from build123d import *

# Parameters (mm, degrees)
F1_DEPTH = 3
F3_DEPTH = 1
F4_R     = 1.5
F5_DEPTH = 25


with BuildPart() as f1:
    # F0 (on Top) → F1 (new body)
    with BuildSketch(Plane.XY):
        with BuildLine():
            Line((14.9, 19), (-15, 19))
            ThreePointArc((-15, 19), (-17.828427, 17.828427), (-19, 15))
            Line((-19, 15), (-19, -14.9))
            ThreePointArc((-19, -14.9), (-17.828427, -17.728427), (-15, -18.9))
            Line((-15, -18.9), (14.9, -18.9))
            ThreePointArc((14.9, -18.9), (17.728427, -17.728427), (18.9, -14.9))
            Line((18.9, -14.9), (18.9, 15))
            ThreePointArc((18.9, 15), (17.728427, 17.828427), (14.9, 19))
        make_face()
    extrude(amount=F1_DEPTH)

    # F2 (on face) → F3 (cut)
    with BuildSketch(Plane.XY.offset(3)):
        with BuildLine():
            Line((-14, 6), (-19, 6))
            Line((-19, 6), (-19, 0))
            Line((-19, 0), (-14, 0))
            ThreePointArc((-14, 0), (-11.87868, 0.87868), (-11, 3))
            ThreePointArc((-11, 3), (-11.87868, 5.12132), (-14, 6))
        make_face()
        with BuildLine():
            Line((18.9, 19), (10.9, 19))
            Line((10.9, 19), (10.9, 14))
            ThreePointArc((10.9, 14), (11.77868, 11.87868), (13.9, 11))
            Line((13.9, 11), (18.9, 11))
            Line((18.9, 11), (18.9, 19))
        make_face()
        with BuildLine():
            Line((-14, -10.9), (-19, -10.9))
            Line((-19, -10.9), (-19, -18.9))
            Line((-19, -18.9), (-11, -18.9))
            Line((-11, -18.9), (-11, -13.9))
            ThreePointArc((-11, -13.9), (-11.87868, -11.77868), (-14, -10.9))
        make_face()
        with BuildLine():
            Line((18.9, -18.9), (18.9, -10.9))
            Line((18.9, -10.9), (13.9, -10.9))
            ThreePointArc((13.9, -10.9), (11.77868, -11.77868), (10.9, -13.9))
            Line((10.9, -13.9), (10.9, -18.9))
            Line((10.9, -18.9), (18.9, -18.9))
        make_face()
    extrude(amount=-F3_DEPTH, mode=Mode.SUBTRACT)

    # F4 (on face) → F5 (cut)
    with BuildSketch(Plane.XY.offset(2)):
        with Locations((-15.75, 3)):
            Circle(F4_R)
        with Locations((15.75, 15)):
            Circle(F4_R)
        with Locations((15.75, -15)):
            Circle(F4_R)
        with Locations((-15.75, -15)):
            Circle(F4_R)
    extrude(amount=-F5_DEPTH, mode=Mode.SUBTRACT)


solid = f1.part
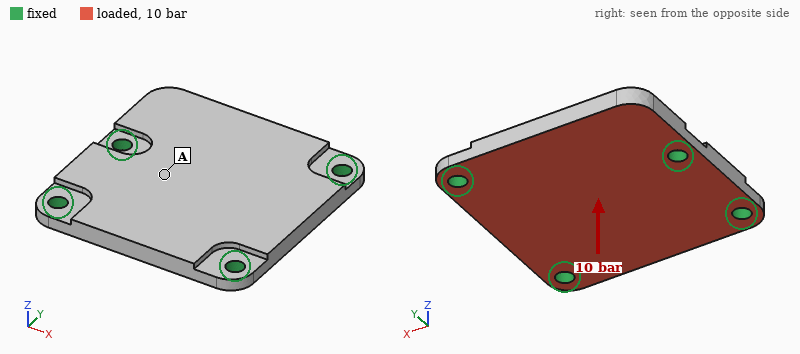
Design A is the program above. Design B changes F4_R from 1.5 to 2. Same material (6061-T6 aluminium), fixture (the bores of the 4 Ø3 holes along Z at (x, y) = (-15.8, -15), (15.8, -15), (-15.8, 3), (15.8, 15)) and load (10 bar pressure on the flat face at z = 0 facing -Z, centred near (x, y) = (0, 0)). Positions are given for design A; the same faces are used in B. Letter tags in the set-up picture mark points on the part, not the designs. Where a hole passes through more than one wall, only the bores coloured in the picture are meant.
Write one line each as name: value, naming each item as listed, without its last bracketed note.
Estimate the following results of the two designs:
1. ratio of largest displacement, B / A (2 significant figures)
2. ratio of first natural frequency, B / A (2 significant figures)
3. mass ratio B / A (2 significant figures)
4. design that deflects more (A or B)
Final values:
ratio of largest displacement, B / A: 0.85
ratio of first natural frequency, B / A: 1.1
mass ratio B / A: 0.99
design that deflects more: A
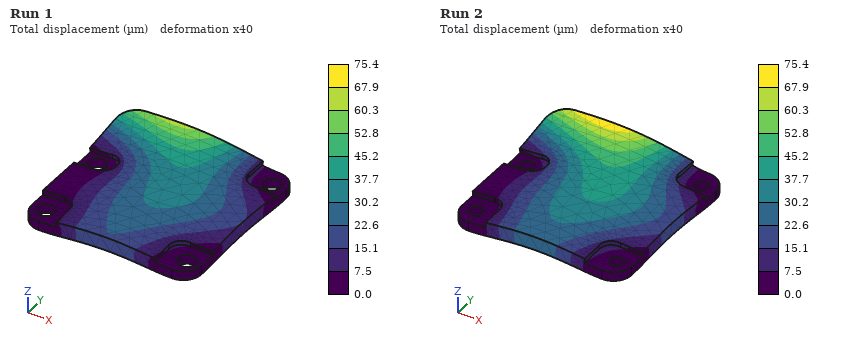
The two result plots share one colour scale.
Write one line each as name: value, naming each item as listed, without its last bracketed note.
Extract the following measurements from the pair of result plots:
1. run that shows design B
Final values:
run that shows design B: Run 1
